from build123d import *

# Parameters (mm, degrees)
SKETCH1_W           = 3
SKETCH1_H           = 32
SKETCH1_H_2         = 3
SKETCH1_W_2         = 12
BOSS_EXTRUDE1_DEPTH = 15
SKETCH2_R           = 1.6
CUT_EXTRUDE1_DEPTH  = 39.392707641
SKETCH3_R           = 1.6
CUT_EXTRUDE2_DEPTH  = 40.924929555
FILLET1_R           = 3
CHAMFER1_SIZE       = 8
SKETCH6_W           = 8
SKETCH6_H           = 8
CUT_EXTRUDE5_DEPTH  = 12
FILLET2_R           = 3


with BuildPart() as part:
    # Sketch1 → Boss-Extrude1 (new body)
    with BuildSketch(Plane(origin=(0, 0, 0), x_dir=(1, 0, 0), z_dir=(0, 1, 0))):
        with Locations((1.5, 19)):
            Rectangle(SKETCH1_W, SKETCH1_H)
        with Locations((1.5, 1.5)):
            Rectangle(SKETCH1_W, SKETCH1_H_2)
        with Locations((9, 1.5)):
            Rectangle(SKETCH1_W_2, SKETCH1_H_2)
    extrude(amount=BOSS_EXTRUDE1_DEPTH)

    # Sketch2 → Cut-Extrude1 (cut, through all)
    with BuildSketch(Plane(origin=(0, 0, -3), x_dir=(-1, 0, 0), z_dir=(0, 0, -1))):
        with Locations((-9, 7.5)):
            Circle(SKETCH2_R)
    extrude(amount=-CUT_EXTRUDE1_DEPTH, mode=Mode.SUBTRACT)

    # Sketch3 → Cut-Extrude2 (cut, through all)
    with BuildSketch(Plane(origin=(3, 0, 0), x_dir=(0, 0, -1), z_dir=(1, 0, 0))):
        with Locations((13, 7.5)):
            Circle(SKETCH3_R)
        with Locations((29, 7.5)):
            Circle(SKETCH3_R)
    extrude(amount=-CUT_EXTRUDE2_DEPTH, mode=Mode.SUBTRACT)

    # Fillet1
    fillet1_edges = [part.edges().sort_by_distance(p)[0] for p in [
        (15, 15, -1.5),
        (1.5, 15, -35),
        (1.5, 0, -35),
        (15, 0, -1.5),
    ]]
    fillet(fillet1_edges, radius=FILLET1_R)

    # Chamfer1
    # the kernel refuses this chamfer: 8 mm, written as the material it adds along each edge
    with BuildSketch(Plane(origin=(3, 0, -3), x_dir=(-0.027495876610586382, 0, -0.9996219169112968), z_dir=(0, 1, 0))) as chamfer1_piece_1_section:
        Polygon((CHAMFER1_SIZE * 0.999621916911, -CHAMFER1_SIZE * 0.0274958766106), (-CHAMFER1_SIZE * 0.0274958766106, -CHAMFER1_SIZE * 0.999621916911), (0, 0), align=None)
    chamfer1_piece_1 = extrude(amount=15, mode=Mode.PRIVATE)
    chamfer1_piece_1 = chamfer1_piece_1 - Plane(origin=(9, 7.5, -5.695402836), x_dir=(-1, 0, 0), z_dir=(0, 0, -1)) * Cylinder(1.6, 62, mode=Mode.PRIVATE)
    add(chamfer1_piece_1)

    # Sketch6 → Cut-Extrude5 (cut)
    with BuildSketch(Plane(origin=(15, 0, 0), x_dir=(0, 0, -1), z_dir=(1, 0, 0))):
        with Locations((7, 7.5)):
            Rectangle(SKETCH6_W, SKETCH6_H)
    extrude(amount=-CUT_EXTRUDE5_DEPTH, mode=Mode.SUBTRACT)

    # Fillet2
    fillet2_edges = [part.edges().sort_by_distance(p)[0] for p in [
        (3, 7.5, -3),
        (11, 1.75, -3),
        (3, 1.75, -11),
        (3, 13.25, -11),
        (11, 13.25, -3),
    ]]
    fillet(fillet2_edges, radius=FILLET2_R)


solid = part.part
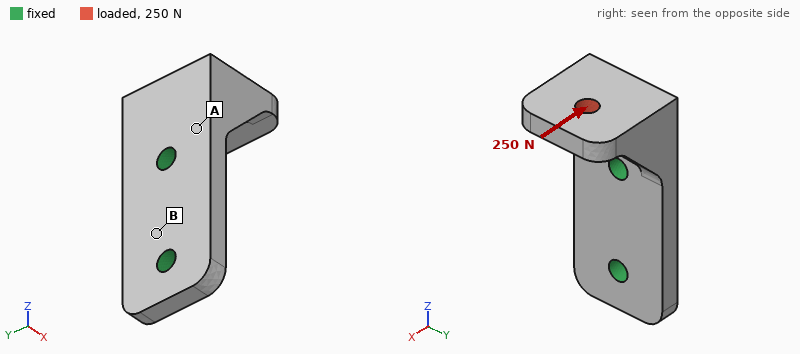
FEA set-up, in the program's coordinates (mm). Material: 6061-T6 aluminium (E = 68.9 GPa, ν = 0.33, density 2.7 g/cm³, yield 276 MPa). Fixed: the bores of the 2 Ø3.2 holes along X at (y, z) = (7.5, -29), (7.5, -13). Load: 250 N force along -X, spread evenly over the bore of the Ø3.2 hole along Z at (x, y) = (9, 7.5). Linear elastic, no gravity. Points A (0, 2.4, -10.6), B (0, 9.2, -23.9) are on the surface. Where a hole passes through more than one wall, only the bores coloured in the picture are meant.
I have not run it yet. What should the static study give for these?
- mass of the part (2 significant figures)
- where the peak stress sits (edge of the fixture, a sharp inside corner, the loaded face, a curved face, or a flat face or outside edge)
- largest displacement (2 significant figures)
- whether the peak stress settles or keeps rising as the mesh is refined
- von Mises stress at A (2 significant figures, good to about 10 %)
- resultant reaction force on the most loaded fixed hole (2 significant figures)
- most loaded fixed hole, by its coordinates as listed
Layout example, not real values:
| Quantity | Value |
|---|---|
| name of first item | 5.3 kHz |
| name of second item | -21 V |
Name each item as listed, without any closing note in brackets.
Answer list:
| Quantity | Value |
|---|---|
| mass of the part | 6.1 g |
| where the peak stress sits | edge of the fixture |
| largest displacement | 77 µm |
| whether the peak stress settles or keeps rising as the mesh is refined | keeps rising |
| von Mises stress at A | 63 MPa |
| resultant reaction force on the most loaded fixed hole | 290 N |
| most loaded fixed hole, by its coordinates as listed | (7.5, -13) |
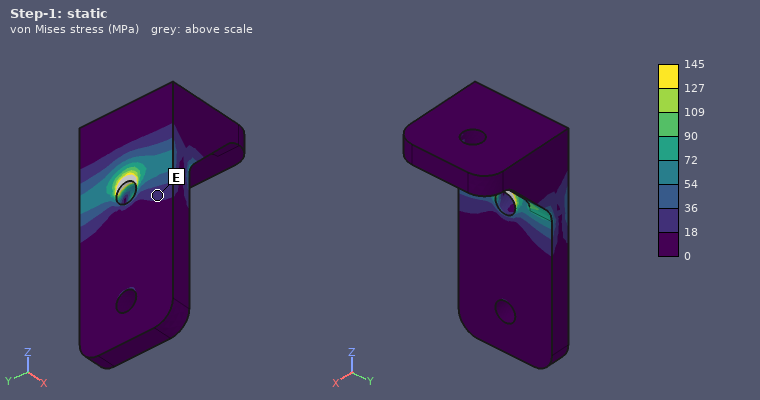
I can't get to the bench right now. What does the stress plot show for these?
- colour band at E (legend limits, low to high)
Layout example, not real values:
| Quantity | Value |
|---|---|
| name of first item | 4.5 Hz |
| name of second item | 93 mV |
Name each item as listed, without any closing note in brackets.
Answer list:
| Quantity | Value |
|---|---|
| colour band at E | 18 to 36 MPa |
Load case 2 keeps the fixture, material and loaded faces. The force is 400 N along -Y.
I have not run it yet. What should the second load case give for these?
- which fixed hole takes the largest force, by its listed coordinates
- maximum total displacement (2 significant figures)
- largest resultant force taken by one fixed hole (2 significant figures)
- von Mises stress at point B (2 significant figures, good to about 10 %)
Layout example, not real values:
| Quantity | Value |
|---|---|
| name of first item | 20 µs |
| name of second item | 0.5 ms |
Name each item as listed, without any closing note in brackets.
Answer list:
| Quantity | Value |
|---|---|
| which fixed hole takes the largest force, by its listed coordinates | (7.5, -13) |
| maximum total displacement | 77 µm |
| largest resultant force taken by one fixed hole | 590 N |
| von Mises stress at point B | 17 MPa |
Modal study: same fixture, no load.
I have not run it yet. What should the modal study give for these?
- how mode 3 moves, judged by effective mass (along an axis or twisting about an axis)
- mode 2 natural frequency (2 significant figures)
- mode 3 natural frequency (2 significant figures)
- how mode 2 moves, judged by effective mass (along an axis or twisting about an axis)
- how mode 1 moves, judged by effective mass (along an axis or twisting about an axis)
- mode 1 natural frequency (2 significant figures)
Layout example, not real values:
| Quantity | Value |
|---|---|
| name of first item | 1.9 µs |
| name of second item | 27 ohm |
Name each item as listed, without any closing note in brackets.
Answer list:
| Quantity | Value |
|---|---|
| how mode 3 moves, judged by effective mass | along Y |
| mode 2 natural frequency | 9500 Hz |
| mode 3 natural frequency | 20 kHz |
| how mode 2 moves, judged by effective mass | along Y |
| how mode 1 moves, judged by effective mass | along X |
| mode 1 natural frequency | 6700 Hz |
